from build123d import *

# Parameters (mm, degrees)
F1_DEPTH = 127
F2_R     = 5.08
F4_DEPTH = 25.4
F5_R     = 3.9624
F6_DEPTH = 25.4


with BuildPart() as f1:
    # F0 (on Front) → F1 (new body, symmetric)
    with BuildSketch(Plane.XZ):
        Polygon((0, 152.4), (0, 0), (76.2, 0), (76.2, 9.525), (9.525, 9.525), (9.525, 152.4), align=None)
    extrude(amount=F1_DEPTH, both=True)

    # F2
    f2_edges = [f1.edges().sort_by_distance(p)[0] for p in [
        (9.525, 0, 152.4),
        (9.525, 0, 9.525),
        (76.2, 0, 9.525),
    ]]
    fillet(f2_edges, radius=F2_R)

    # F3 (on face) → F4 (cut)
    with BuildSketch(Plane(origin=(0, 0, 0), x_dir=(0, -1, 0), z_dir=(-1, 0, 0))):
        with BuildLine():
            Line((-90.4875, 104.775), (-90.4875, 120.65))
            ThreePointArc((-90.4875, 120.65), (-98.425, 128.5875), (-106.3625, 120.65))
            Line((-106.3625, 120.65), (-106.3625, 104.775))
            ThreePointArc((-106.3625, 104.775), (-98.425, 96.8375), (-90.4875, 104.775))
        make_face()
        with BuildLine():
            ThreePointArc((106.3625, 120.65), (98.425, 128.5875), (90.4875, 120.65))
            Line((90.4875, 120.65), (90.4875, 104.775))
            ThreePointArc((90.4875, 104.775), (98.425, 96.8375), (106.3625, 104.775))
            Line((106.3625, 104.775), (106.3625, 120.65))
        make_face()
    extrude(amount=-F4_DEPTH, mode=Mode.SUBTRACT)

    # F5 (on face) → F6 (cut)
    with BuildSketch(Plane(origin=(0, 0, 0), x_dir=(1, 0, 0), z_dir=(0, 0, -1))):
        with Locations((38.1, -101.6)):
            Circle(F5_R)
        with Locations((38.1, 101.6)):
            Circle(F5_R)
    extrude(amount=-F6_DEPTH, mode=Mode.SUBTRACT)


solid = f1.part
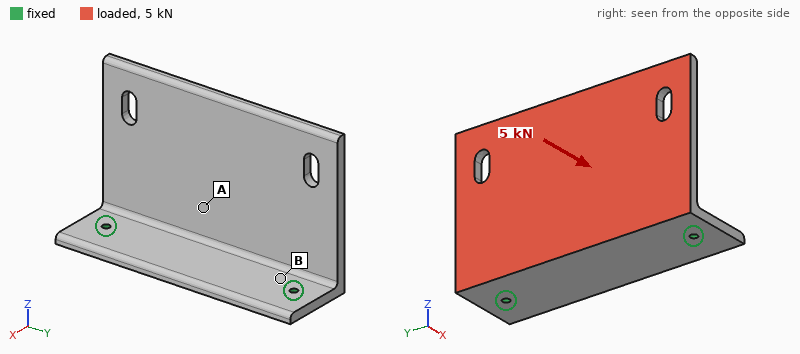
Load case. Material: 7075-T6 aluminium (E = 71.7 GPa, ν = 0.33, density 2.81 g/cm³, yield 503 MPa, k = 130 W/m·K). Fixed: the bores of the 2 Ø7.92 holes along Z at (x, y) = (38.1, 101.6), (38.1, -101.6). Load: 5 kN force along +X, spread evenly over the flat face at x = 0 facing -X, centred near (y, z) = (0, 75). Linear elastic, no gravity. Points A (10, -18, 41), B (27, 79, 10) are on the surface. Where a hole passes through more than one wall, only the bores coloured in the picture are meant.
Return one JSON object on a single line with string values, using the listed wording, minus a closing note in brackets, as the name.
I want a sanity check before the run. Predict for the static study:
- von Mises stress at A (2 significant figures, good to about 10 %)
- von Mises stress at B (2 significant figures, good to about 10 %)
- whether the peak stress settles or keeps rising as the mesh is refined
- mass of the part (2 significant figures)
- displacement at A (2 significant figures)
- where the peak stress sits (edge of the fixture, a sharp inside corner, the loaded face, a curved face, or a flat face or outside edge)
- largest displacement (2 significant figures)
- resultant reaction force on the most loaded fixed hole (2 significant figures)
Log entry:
{"von Mises stress at A": "44 MPa", "von Mises stress at B": "96 MPa", "whether the peak stress settles or keeps rising as the mesh is refined": "keeps rising", "mass of the part": "1.5 kg", "displacement at A": "0.69 mm", "where the peak stress sits": "edge of the fixture", "largest displacement": "3.4 mm", "resultant reaction force on the most loaded fixed hole": "2.6 kN"}
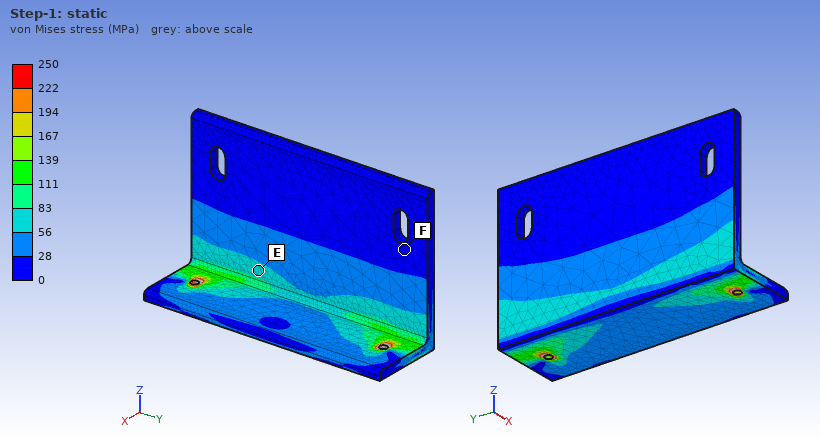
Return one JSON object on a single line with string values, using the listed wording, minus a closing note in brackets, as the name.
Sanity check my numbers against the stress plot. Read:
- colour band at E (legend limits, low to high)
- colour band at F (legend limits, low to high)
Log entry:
{"colour band at E": "56 to 83 MPa", "colour band at F": "0 to 28 MPa"}
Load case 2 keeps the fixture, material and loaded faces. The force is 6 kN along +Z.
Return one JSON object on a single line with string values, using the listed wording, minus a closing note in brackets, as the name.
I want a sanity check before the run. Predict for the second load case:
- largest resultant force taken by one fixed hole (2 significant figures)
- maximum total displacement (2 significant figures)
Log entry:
{"largest resultant force taken by one fixed hole": "3.0 kN", "maximum total displacement": "1.1 mm"}
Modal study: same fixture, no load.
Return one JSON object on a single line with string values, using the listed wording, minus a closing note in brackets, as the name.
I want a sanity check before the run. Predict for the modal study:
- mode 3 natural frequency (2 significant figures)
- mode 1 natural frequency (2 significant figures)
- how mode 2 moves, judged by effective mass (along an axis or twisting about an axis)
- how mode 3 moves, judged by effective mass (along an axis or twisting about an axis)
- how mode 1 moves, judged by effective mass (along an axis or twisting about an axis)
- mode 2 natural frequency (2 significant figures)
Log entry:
{"mode 3 natural frequency": "1100 Hz", "mode 1 natural frequency": "240 Hz", "how mode 2 moves, judged by effective mass": "twisting about Z", "how mode 3 moves, judged by effective mass": "along Z", "how mode 1 moves, judged by effective mass": "along X", "mode 2 natural frequency": "520 Hz"}
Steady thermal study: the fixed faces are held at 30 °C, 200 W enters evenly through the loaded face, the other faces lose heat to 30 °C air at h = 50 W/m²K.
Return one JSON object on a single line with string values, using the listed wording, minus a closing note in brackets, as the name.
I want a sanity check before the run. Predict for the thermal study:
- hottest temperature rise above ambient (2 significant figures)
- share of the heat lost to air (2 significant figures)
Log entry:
{"hottest temperature rise above ambient": "47 K", "share of the heat lost to air": "55 %"}
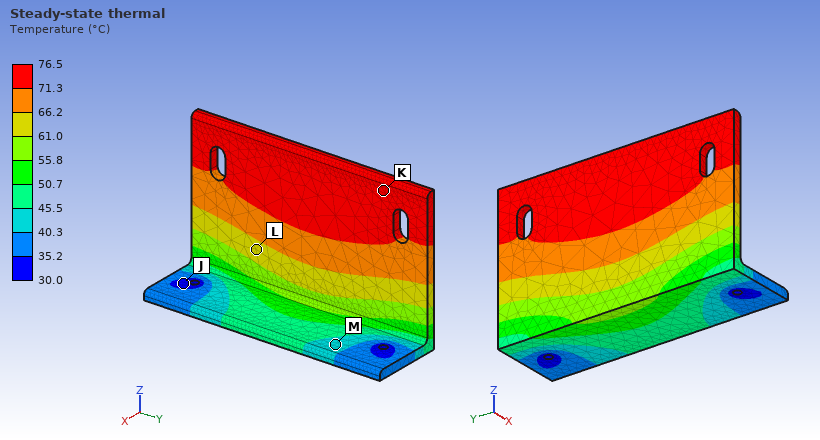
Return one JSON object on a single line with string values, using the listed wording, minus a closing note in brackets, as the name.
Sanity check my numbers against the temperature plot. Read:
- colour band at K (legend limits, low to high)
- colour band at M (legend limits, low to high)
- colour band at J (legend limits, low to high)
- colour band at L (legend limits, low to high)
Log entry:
{"colour band at K": "71.3 to 76.5 °C", "colour band at M": "40.3 to 45.5 °C", "colour band at J": "30.0 to 35.2 °C", "colour band at L": "61.0 to 66.2 °C"}
